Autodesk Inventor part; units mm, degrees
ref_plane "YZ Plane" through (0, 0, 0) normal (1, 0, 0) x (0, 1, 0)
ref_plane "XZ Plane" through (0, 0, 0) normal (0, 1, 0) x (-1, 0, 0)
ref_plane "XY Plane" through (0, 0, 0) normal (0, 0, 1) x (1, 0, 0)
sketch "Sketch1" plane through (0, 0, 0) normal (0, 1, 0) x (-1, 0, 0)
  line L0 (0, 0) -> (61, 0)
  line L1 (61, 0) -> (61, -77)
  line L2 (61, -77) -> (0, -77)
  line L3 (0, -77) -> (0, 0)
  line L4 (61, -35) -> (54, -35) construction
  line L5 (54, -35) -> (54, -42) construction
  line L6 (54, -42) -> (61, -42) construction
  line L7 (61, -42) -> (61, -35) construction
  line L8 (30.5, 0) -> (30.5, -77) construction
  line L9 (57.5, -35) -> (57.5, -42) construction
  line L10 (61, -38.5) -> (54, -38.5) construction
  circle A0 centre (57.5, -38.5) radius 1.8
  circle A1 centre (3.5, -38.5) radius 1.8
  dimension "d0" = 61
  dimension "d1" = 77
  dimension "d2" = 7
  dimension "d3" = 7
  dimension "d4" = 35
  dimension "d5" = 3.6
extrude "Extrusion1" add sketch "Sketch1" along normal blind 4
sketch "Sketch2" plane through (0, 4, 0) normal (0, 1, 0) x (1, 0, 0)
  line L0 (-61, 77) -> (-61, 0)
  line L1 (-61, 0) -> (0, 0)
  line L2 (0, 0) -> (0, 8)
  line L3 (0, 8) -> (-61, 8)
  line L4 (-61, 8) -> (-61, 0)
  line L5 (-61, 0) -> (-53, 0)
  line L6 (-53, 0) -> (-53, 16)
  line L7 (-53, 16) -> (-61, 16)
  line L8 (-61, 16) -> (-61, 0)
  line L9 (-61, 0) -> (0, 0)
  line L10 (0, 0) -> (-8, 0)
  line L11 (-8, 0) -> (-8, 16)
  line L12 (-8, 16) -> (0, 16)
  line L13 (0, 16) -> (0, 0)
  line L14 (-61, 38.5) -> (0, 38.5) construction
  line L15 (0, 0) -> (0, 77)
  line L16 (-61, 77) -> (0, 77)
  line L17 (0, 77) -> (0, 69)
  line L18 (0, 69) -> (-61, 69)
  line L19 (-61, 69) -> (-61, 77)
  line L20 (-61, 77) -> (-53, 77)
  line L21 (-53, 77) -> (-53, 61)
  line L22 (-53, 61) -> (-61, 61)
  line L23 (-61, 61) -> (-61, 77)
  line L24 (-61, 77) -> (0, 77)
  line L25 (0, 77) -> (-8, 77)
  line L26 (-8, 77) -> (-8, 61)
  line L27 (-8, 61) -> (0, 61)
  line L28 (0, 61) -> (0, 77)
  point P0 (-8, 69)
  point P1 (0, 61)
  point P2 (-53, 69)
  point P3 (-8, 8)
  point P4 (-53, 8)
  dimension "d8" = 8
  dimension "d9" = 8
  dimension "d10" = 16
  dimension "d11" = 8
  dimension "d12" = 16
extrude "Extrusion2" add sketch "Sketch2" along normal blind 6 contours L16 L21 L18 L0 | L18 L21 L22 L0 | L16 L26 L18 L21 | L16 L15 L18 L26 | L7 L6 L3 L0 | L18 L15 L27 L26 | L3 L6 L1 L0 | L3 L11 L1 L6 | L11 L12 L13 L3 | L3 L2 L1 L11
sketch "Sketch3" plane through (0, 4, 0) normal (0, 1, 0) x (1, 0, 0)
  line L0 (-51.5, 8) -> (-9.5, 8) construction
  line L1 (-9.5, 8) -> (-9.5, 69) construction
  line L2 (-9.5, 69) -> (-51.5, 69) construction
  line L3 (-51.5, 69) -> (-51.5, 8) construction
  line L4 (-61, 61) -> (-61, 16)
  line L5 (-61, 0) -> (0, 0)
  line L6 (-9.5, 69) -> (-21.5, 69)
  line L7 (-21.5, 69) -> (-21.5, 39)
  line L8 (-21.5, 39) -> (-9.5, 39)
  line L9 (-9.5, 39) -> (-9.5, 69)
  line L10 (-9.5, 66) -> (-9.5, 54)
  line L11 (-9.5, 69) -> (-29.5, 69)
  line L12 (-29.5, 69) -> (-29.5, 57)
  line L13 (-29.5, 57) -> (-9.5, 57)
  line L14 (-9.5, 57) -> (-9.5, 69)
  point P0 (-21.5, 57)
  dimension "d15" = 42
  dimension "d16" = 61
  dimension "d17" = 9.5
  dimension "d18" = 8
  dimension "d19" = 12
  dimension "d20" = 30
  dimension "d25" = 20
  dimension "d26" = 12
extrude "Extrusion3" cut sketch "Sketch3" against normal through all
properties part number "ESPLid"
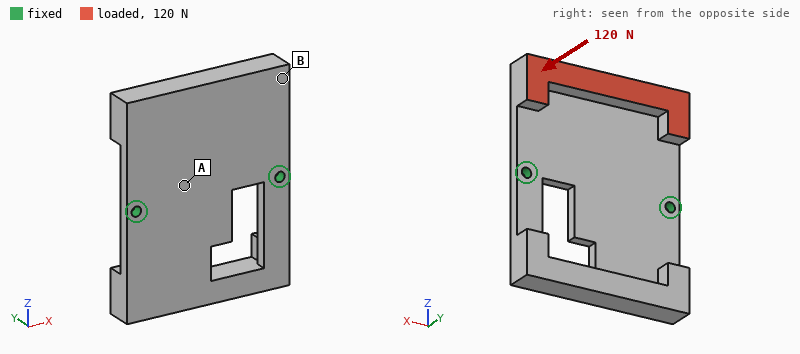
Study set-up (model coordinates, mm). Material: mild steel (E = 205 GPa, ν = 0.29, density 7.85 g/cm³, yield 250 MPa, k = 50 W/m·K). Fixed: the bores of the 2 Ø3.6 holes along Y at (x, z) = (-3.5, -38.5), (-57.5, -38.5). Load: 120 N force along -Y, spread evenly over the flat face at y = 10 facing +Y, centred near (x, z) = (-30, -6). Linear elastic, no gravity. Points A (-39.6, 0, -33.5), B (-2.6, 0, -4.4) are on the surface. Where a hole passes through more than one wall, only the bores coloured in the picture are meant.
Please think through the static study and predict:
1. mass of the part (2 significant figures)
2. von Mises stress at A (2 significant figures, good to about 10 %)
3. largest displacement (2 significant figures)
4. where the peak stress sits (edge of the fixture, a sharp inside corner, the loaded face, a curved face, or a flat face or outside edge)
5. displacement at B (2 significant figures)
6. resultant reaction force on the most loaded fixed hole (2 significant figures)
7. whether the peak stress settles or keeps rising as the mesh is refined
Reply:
190 g
13 MPa
42 µm
edge of the fixture
34 µm
64 N
keeps rising
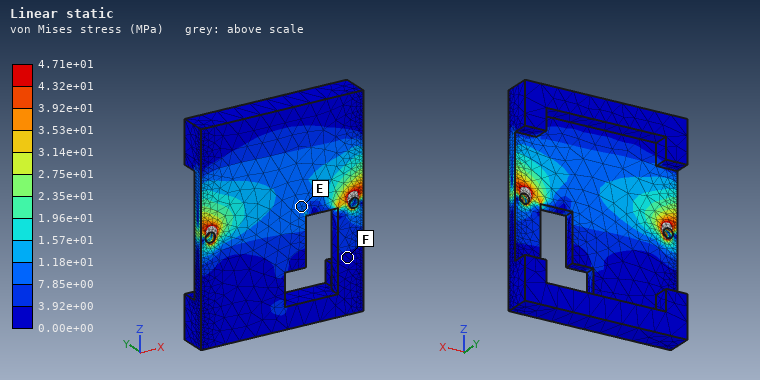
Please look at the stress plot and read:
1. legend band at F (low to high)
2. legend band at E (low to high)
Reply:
0.00e+00 to 3.92e+00 MPa
7.85e+00 to 1.18e+01 MPa
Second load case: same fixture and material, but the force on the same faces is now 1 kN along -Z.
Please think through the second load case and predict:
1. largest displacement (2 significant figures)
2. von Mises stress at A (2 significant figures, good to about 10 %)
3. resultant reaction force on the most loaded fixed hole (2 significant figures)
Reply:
0.12 mm
33 MPa
520 N
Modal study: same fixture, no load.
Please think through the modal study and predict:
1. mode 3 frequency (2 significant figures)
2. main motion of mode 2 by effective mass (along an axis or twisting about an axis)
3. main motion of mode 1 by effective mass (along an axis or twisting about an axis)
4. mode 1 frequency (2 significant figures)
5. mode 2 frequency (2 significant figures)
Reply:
3100 Hz
along Y
twisting about X
1100 Hz
1400 Hz
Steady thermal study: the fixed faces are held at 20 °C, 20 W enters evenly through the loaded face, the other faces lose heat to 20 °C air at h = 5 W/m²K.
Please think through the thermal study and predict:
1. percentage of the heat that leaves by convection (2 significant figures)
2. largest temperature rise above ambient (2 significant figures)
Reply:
8.6 %
68 K
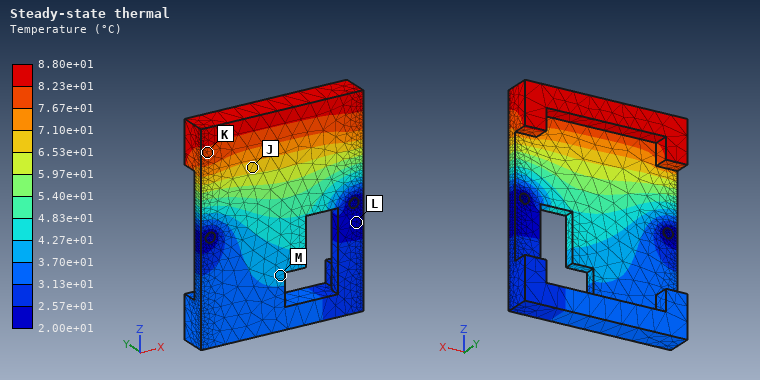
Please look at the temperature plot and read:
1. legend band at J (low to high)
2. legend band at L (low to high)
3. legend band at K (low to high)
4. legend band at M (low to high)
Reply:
6.53e+01 to 7.10e+01 °C
2.00e+01 to 2.57e+01 °C
7.67e+01 to 8.23e+01 °C
3.70e+01 to 4.27e+01 °C
